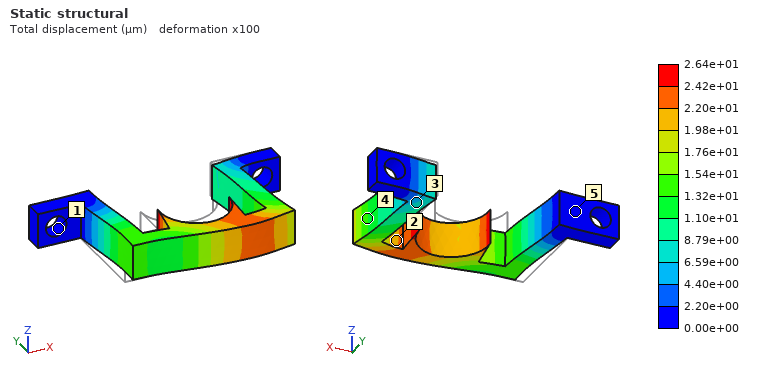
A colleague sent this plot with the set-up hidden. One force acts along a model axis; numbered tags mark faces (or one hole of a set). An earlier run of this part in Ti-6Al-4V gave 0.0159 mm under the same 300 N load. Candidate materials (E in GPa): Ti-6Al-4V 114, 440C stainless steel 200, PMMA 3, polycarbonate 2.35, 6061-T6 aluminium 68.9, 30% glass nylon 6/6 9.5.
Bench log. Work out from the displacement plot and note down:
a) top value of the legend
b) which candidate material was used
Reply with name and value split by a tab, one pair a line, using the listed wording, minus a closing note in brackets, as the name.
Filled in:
top value of the legend	2.64e+01 µm
which candidate material was used	6061-T6 aluminium
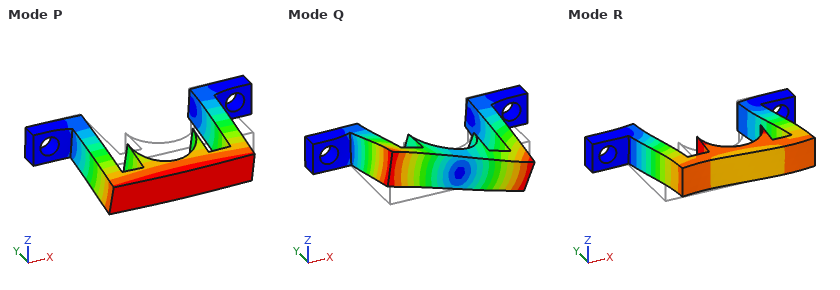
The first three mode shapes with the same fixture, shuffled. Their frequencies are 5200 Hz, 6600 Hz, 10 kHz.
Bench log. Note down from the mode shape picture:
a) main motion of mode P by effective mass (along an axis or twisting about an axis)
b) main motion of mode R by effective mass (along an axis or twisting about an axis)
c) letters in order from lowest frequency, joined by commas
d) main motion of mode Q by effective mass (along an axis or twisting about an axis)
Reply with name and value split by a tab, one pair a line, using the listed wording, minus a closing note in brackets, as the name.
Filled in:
main motion of mode P by effective mass	along Z
main motion of mode R by effective mass	along X
letters in order from lowest frequency, joined by commas	P, R, Q
main motion of mode Q by effective mass	twisting about Y
